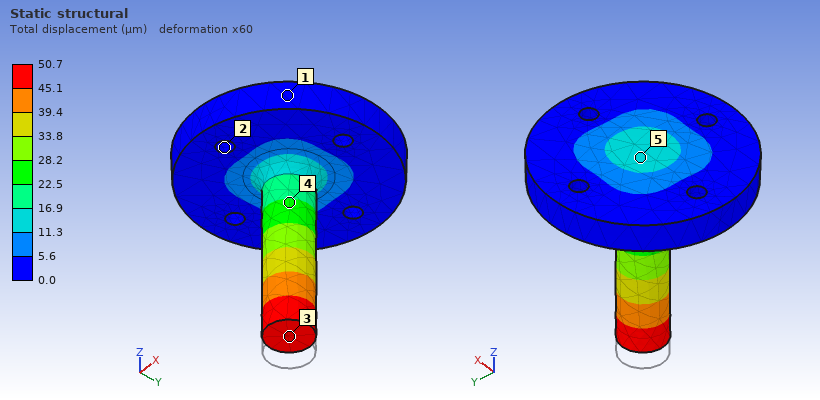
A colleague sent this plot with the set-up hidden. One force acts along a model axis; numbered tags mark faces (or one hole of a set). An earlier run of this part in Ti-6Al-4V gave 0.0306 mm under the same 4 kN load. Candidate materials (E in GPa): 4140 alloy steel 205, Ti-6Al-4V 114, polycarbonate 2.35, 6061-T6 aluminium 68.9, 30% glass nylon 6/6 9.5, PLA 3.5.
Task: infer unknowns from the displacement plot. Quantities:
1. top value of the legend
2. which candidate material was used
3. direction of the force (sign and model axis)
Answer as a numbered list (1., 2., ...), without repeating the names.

1. 50.7 µm
2. 6061-T6 aluminium
3. +Z
